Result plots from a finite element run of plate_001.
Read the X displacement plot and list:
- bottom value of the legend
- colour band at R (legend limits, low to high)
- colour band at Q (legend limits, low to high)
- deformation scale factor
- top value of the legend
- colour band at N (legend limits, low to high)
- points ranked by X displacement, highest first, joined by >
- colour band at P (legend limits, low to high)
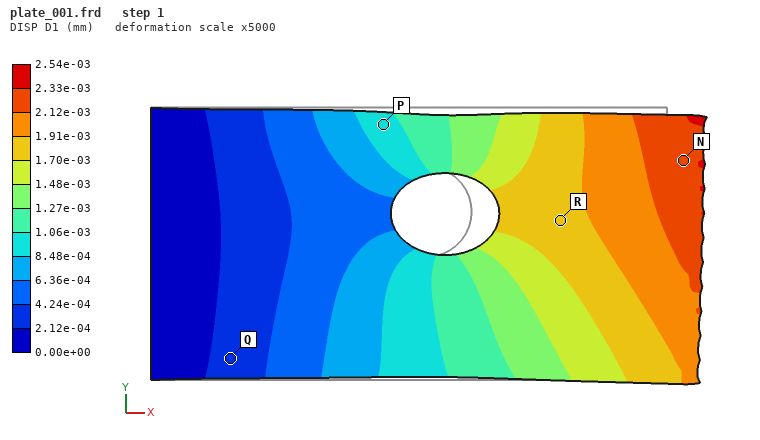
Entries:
0.00e+00 mm
1.70e-03 to 1.91e-03 mm
2.12e-04 to 4.24e-04 mm
5000
2.54e-03 mm
2.12e-03 to 2.33e-03 mm
N > R > P > Q
8.48e-04 to 1.06e-03 mm
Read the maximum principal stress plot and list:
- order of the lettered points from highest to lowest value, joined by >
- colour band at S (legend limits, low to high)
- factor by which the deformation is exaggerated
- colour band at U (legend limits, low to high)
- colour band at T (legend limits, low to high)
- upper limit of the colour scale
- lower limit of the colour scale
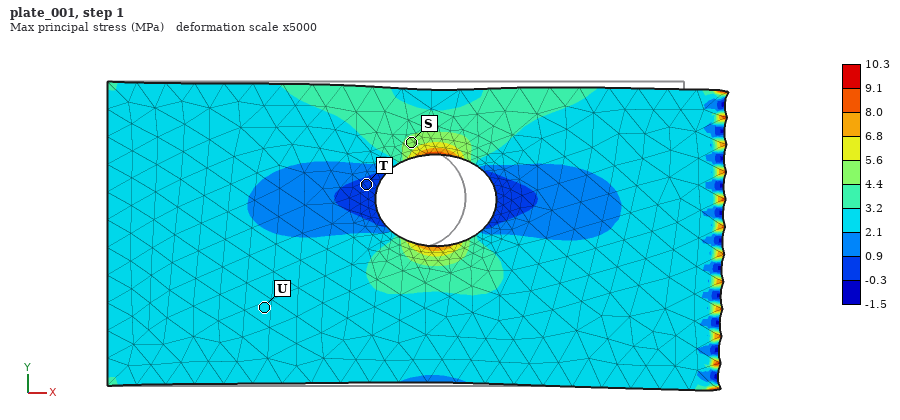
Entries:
S > U > T
4.4 to 5.6 MPa
5000
2.1 to 3.2 MPa
-0.3 to 0.9 MPa
10.3 MPa
-1.5 MPa
